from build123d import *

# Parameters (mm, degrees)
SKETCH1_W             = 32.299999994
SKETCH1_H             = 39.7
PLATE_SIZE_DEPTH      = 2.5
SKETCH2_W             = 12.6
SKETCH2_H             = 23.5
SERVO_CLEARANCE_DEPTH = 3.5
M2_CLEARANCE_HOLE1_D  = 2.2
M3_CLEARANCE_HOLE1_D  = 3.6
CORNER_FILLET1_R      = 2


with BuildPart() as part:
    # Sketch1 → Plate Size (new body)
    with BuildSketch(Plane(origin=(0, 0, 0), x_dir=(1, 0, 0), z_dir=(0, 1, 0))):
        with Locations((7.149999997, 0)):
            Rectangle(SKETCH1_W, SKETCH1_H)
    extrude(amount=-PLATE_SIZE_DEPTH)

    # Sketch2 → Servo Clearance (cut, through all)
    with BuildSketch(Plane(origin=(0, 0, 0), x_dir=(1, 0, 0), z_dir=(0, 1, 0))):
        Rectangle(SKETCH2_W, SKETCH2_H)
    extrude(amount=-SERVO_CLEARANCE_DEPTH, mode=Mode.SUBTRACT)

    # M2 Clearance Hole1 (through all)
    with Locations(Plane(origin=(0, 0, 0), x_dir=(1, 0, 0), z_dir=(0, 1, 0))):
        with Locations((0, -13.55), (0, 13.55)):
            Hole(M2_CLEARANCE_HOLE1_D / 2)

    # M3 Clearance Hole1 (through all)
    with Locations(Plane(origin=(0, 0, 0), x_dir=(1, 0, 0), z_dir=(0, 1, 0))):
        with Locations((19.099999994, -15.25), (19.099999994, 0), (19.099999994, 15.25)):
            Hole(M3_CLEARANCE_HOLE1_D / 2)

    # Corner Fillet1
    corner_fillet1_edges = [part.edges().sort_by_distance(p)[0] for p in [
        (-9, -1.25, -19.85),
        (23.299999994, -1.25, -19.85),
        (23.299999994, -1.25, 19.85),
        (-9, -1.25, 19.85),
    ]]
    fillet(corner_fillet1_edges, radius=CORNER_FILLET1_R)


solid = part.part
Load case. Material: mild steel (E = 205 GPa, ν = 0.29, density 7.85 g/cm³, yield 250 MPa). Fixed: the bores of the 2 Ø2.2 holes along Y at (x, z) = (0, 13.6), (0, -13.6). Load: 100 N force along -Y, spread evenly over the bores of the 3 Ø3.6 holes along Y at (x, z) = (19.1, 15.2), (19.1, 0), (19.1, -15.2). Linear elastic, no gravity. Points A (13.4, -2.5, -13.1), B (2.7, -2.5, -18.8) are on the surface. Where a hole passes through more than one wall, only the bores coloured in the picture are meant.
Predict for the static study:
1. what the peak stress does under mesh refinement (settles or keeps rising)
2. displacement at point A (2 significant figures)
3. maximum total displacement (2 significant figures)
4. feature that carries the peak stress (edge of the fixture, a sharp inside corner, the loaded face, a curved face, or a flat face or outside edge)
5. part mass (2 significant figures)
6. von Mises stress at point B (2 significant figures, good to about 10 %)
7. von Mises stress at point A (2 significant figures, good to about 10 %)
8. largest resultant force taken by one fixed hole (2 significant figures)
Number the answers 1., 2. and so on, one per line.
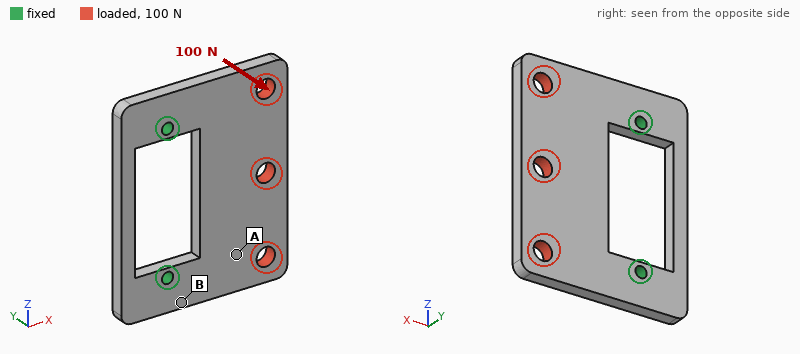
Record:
1. keeps rising
2. 31 µm
3. 71 µm
4. edge of the fixture
5. 19 g
6. 70 MPa
7. 18 MPa
8. 50 N
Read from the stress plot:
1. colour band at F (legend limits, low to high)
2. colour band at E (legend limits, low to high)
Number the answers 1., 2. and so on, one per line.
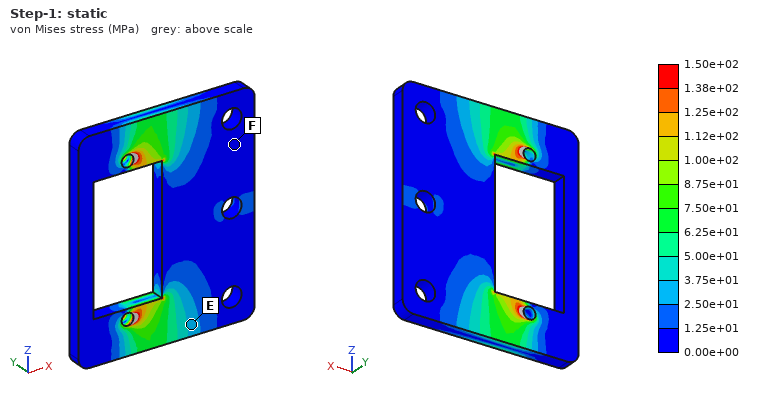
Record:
1. 0.00e+00 to 1.25e+01 MPa
2. 2.50e+01 to 3.75e+01 MPa
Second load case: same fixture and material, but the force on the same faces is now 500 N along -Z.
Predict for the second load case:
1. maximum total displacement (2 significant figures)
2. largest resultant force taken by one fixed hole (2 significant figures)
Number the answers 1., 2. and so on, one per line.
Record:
1. 7.9 µm
2. 360 N
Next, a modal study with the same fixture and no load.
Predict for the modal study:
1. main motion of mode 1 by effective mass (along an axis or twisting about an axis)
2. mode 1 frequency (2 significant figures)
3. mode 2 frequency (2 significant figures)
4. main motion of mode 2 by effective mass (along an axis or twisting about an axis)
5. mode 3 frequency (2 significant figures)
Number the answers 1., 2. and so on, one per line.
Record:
1. along Y
2. 2500 Hz
3. 5800 Hz
4. twisting about X
5. 10 kHz
